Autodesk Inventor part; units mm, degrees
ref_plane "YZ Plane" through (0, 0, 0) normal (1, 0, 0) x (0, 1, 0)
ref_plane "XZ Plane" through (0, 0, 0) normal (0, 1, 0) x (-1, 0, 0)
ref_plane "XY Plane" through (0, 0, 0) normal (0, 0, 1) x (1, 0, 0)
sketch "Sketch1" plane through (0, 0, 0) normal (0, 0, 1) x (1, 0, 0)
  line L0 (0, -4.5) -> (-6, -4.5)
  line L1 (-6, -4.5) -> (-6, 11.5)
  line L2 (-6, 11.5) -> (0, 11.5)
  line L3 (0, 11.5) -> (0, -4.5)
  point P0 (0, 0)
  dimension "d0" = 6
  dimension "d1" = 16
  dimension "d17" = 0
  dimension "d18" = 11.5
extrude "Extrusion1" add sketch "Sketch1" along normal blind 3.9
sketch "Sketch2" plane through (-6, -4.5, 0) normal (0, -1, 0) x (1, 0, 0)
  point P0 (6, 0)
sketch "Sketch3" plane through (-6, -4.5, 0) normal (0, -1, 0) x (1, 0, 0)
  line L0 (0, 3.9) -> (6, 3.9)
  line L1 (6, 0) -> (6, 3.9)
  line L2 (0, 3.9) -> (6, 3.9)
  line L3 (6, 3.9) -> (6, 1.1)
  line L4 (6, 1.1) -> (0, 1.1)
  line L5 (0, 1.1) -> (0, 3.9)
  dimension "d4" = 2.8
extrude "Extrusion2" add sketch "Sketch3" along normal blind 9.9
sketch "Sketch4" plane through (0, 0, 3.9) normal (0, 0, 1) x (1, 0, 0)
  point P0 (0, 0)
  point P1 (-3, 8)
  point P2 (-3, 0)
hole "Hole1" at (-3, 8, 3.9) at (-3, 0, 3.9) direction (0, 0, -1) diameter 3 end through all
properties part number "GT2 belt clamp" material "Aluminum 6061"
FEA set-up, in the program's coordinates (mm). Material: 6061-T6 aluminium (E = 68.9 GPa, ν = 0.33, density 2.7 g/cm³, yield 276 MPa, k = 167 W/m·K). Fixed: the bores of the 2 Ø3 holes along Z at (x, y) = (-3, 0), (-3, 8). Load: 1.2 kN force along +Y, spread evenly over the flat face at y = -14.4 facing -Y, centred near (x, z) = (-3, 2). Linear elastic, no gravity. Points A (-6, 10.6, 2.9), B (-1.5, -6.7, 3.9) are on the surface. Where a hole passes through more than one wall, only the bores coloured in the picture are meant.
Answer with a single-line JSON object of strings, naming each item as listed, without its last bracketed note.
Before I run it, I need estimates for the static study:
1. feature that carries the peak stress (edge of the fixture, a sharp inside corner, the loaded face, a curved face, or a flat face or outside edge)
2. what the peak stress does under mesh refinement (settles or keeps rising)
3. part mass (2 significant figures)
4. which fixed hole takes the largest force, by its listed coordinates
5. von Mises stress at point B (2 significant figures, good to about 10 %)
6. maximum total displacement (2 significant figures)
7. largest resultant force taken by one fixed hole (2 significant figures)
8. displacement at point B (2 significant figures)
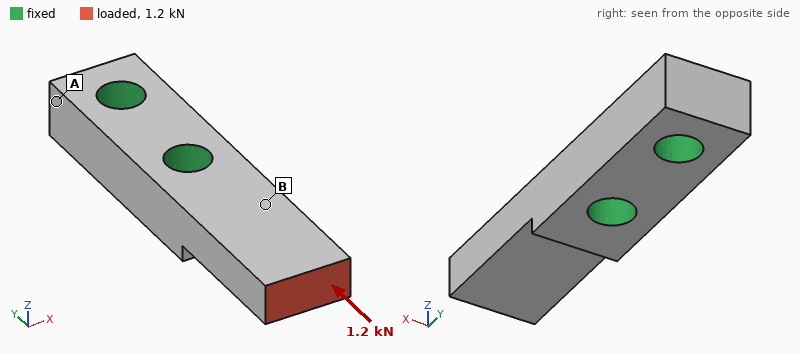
{"feature that carries the peak stress": "edge of the fixture", "what the peak stress does under mesh refinement": "keeps rising", "part mass": "1.3 g", "which fixed hole takes the largest force, by its listed coordinates": "(-3, 0)", "von Mises stress at point B": "72 MPa", "maximum total displacement": "19 µm", "largest resultant force taken by one fixed hole": "1.2 kN", "displacement at point B": "8.6 µm"}
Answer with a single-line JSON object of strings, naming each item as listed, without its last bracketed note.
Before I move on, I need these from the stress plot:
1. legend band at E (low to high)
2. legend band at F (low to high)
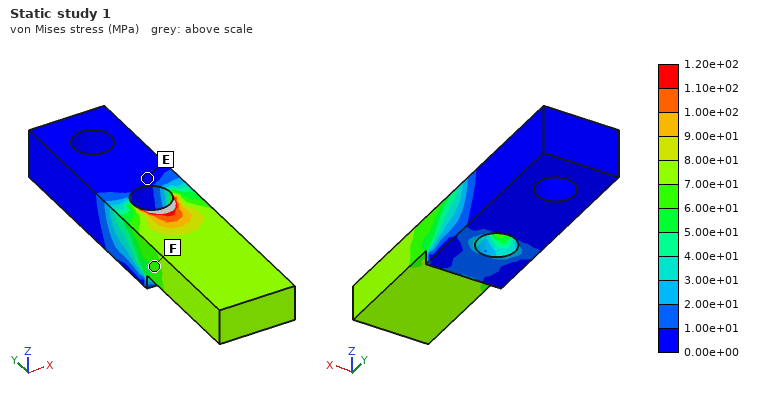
{"legend band at E": "0.00e+00 to 1.00e+01 MPa", "legend band at F": "6.00e+01 to 7.00e+01 MPa"}
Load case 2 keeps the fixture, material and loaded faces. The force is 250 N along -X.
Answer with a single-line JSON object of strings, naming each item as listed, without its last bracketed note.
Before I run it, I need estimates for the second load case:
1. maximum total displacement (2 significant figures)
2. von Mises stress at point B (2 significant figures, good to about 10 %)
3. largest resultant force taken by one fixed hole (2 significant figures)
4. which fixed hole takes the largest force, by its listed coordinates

{"maximum total displacement": "77 µm", "von Mises stress at point B": "59 MPa", "largest resultant force taken by one fixed hole": "330 N", "which fixed hole takes the largest force, by its listed coordinates": "(-3, 0)"}
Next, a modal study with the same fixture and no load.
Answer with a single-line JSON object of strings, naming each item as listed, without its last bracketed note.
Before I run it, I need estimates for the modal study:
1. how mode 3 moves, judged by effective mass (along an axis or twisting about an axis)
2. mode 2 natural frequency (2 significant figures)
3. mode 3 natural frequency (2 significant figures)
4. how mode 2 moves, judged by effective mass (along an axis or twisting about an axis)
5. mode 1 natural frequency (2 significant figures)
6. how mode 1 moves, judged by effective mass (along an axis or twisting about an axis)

{"how mode 3 moves, judged by effective mass": "twisting about Y", "mode 2 natural frequency": "23 kHz", "mode 3 natural frequency": "48 kHz", "how mode 2 moves, judged by effective mass": "along X", "mode 1 natural frequency": "15 kHz", "how mode 1 moves, judged by effective mass": "along Z"}
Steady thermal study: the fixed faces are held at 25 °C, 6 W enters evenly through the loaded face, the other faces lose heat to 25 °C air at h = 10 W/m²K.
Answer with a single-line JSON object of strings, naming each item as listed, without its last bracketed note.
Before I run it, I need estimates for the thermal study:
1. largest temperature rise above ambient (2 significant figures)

{"largest temperature rise above ambient": "27 K"}
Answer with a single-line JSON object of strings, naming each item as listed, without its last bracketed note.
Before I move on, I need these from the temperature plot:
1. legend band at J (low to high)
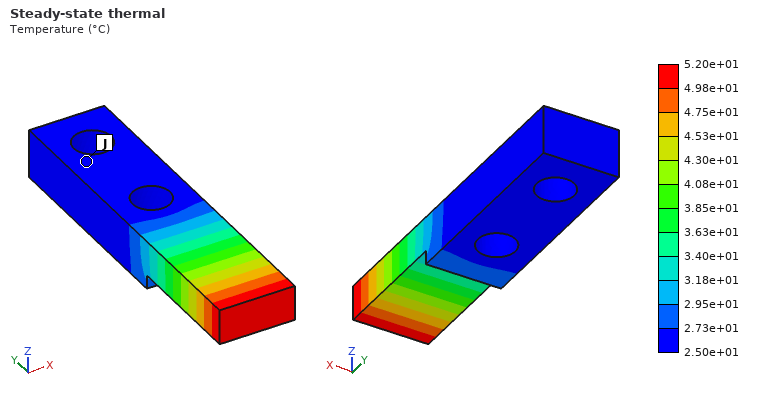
{"legend band at J": "2.50e+01 to 2.73e+01 °C"}
